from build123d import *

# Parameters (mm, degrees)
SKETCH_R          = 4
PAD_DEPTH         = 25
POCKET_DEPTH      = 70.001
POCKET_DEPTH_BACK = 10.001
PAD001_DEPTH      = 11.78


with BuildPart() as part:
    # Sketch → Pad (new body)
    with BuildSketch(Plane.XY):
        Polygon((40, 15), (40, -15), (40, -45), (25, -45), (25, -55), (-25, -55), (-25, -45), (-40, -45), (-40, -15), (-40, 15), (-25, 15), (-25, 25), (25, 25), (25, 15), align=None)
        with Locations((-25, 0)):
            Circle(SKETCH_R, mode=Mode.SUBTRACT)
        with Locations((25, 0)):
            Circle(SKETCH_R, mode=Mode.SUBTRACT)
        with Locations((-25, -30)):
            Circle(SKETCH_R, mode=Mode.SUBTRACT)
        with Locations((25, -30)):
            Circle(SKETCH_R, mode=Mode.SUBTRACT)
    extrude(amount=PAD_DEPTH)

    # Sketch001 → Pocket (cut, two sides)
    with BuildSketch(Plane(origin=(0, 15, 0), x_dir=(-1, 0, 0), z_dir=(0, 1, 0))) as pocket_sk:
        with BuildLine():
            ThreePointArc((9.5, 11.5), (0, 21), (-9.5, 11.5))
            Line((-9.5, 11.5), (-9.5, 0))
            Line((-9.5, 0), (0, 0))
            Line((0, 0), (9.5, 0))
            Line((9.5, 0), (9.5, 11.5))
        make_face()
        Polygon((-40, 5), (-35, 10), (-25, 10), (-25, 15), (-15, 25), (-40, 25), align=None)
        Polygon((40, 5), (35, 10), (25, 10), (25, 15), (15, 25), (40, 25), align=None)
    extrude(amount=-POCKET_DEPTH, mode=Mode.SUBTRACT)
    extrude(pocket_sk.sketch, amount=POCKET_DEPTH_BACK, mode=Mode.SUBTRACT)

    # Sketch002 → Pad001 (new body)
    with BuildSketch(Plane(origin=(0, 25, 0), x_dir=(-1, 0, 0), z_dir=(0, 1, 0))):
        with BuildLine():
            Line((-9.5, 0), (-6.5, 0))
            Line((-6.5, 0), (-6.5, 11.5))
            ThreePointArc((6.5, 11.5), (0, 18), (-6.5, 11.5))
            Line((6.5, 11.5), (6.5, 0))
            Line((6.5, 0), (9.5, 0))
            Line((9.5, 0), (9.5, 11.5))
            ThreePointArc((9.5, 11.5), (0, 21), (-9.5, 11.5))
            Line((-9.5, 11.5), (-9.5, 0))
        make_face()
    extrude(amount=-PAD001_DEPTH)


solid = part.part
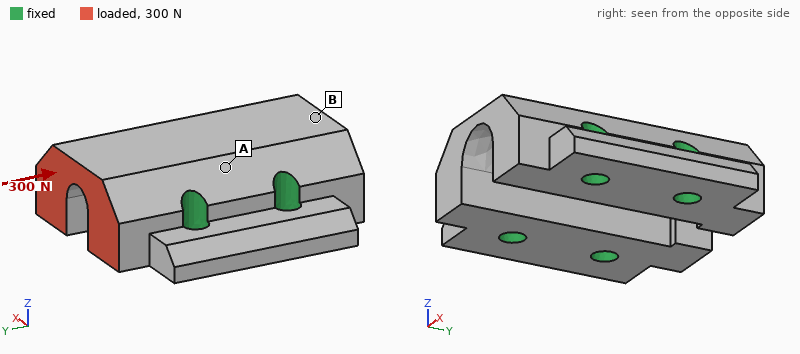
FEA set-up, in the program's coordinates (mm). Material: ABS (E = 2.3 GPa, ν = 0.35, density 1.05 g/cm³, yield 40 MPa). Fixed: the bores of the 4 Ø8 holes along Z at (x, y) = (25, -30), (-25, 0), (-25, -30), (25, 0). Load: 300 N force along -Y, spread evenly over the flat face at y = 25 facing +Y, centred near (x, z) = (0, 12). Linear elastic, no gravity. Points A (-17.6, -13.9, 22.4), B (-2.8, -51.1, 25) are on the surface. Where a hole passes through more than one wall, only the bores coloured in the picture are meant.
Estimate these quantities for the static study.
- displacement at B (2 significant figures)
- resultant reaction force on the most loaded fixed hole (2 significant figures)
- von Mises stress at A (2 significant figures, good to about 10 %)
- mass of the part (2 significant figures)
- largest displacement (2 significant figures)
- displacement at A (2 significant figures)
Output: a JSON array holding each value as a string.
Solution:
["2.0 µm", "110 N", "0.23 MPa", "83 g", "10 µm", "1.9 µm"]
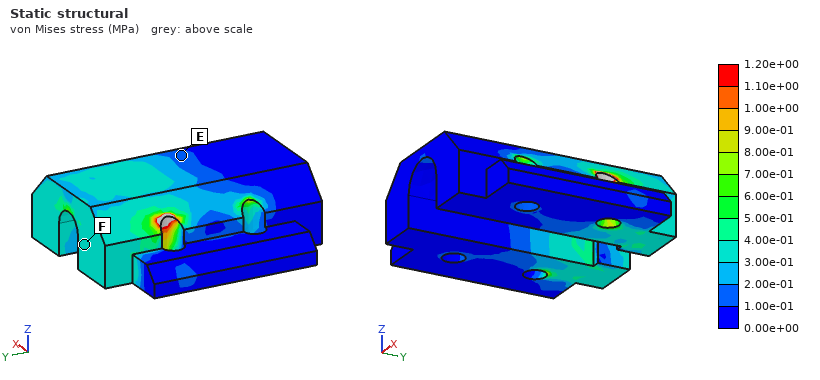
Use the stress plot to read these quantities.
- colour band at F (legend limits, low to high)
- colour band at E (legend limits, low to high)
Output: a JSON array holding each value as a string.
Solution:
["3.00e-01 to 4.00e-01 MPa", "1.00e-01 to 2.00e-01 MPa"]
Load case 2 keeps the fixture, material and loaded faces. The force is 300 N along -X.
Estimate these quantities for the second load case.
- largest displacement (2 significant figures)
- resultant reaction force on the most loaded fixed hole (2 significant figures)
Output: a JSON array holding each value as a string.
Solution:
["38 µm", "200 N"]
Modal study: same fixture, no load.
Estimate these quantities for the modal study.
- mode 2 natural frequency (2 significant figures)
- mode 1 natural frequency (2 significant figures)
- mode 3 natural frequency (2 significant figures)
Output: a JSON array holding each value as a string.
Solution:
["5000 Hz", "4400 Hz", "5000 Hz"]
